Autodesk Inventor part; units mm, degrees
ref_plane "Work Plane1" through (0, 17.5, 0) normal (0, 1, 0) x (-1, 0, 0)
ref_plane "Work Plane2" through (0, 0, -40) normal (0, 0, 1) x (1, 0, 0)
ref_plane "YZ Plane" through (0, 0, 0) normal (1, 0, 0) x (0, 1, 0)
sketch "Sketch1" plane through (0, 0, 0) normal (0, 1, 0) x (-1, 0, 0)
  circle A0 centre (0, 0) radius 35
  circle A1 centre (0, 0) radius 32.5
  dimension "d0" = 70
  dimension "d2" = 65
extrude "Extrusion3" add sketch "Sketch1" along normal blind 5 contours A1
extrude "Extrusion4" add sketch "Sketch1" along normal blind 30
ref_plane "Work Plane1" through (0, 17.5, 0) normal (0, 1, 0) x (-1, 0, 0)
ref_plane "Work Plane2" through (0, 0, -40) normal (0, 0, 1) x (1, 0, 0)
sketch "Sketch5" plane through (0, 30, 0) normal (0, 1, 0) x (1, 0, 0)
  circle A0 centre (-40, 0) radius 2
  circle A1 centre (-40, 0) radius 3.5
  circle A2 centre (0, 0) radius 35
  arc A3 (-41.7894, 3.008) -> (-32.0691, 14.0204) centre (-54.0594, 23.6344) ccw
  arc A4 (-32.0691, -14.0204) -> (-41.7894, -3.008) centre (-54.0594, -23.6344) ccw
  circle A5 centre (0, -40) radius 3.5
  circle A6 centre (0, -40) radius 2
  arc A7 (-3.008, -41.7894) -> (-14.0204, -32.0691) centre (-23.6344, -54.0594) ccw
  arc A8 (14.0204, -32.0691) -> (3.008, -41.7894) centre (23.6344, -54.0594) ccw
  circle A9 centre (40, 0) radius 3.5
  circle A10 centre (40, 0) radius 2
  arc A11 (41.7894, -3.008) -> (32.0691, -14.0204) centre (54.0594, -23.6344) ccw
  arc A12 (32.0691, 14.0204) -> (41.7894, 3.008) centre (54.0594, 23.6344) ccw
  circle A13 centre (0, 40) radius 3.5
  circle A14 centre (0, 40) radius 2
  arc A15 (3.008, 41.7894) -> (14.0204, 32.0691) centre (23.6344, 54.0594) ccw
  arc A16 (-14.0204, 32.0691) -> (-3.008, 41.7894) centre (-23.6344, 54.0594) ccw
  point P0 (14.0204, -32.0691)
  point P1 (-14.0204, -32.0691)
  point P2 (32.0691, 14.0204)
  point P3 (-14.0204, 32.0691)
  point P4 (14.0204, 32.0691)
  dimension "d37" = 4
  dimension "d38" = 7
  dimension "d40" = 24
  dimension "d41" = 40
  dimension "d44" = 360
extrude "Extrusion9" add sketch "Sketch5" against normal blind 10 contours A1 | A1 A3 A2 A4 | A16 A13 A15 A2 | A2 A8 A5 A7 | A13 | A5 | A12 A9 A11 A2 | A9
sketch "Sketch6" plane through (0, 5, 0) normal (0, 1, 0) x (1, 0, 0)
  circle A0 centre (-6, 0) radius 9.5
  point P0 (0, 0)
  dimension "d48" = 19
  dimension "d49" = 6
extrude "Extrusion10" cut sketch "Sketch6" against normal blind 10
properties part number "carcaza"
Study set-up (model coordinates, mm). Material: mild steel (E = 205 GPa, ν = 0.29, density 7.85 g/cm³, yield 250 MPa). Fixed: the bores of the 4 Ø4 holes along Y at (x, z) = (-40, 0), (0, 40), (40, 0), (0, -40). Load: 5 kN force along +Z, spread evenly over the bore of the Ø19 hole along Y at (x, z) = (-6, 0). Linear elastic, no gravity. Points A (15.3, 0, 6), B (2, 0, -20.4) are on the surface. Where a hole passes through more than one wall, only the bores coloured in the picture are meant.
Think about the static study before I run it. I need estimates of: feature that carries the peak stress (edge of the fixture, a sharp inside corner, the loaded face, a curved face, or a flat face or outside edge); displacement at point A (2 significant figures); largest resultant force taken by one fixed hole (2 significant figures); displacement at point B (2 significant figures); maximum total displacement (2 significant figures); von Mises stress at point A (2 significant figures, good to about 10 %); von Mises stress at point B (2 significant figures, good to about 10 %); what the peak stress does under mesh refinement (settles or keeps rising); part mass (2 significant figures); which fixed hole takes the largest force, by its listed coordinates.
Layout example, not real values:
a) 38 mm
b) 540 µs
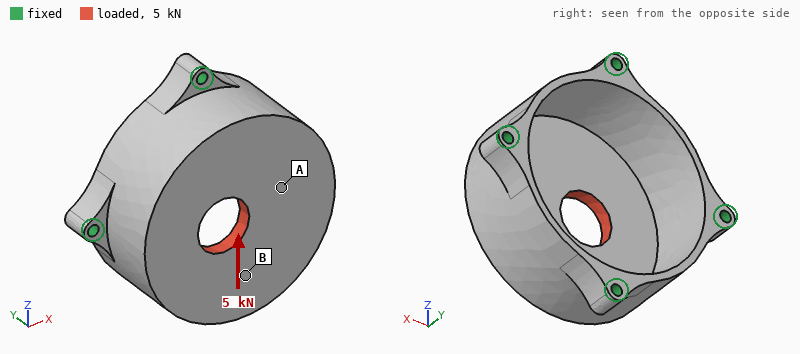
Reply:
a) edge of the fixture
b) 9.9 µm
c) 2.0 kN
d) 11 µm
e) 12 µm
f) 7.6 MPa
g) 18 MPa
h) keeps rising
i) 270 g
j) (-40, 0)
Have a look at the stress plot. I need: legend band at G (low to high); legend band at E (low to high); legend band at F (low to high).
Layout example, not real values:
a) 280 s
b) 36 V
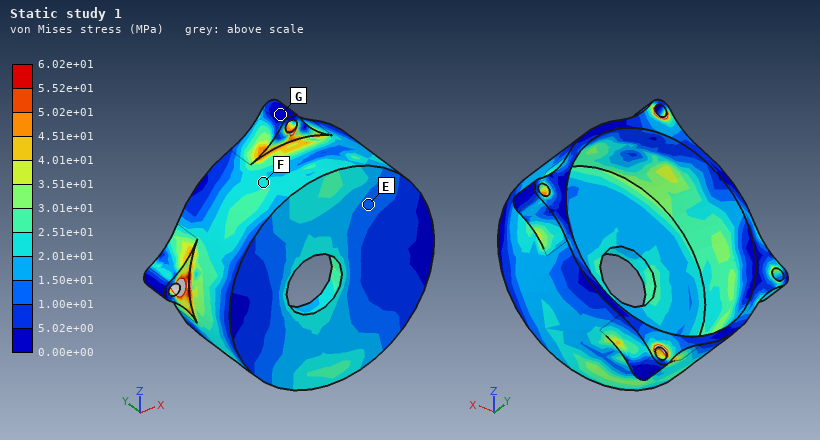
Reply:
a) 0.00e+00 to 5.02e+00 MPa
b) 1.00e+01 to 1.50e+01 MPa
c) 2.01e+01 to 2.51e+01 MPa
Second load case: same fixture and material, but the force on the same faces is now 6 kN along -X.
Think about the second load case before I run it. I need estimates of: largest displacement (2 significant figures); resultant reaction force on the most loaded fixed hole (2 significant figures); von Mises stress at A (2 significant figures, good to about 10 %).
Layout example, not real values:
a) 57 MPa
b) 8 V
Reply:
a) 15 µm
b) 2.1 kN
c) 18 MPa
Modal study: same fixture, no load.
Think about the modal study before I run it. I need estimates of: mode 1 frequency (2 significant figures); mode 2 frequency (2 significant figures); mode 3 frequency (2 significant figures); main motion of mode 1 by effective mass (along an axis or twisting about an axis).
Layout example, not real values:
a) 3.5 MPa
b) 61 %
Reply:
a) 6800 Hz
b) 8700 Hz
c) 8700 Hz
d) along Y
